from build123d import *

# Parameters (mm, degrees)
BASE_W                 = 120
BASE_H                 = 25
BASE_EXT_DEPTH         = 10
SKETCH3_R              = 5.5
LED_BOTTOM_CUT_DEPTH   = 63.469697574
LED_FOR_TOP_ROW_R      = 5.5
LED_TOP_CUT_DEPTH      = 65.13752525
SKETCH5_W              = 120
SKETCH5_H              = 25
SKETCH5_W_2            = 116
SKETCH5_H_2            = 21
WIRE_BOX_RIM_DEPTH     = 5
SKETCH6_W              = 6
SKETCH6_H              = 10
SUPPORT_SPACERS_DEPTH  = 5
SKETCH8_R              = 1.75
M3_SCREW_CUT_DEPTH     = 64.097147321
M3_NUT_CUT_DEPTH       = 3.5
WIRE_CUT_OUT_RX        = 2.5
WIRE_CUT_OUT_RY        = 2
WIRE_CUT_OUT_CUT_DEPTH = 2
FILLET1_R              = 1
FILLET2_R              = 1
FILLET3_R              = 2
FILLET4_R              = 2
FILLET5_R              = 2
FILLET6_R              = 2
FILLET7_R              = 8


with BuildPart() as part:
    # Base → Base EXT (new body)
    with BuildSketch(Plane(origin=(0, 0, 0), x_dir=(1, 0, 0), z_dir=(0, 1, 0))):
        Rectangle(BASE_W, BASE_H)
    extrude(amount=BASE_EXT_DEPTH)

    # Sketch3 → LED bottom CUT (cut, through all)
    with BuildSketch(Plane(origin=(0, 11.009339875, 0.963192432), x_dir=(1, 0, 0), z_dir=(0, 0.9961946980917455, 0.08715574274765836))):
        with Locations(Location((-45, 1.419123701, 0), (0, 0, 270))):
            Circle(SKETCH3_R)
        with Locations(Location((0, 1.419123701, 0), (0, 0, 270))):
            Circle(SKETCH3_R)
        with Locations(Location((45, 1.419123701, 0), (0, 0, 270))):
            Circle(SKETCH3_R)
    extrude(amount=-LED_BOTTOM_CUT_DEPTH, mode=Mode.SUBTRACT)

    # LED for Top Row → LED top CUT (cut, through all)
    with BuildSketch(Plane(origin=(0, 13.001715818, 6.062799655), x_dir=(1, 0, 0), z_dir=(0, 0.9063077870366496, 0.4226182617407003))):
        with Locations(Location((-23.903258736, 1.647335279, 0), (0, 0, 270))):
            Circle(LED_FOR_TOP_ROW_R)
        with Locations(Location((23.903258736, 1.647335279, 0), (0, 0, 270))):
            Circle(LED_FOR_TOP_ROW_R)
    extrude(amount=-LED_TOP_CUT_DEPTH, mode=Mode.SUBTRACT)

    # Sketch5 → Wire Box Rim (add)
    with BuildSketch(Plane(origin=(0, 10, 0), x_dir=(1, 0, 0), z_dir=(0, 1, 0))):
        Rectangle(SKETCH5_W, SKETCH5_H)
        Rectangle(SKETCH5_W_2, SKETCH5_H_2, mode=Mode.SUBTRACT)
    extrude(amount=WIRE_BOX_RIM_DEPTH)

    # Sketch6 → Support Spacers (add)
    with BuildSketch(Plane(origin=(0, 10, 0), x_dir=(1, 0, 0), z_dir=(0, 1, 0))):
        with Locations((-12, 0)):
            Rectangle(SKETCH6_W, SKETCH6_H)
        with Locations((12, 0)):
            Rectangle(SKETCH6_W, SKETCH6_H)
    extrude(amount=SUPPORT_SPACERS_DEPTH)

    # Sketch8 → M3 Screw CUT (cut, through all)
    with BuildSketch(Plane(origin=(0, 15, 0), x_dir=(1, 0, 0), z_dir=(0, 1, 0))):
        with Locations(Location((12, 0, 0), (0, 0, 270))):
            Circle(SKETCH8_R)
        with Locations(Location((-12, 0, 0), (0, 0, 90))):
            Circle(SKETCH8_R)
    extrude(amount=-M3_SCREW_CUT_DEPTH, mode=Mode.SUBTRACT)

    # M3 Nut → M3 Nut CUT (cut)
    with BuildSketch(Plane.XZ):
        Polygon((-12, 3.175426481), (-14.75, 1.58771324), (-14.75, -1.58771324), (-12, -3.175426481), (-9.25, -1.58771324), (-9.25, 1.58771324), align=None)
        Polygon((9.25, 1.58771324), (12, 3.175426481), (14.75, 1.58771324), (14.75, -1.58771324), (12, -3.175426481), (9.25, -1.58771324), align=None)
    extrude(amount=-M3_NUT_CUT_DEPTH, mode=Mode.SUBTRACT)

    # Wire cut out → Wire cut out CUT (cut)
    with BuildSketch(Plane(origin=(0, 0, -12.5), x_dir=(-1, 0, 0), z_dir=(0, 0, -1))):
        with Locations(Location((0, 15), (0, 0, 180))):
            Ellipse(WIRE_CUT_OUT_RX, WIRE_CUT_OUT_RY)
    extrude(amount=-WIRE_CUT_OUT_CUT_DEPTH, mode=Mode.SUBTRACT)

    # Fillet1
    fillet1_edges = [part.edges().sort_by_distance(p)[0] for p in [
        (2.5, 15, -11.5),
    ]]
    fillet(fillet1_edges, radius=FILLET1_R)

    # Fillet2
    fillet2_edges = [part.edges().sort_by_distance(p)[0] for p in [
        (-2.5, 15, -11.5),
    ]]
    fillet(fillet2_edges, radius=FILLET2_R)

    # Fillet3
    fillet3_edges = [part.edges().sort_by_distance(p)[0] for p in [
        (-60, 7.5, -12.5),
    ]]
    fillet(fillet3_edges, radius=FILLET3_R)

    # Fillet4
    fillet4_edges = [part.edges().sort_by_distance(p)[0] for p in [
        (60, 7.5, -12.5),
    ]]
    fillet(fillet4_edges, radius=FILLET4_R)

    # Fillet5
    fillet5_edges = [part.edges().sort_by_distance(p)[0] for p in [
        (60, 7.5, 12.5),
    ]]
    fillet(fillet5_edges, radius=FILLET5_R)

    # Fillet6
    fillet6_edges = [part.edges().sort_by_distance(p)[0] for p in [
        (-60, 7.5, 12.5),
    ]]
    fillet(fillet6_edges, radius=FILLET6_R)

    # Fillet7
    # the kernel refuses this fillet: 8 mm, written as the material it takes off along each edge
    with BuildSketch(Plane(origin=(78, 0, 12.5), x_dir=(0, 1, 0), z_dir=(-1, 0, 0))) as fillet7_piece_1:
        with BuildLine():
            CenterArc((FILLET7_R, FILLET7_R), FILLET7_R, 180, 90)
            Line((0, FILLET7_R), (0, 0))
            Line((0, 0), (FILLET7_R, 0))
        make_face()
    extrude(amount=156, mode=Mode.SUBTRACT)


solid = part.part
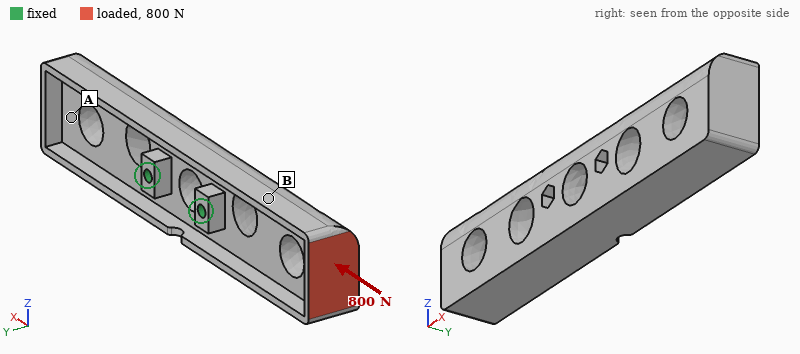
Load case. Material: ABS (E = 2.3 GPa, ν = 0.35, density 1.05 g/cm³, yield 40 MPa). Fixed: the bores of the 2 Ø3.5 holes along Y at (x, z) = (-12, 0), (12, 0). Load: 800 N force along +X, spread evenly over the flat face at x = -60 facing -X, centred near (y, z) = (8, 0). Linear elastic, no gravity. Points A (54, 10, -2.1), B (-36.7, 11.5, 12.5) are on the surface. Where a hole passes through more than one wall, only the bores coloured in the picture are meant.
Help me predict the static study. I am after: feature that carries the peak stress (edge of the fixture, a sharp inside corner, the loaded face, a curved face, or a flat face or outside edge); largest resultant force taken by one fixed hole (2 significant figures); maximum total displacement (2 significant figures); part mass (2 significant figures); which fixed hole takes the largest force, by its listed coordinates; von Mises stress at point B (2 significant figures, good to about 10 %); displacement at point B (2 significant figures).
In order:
the loaded face
560 N
0.65 mm
28 g
(-12, 0)
8.7 MPa
0.16 mm
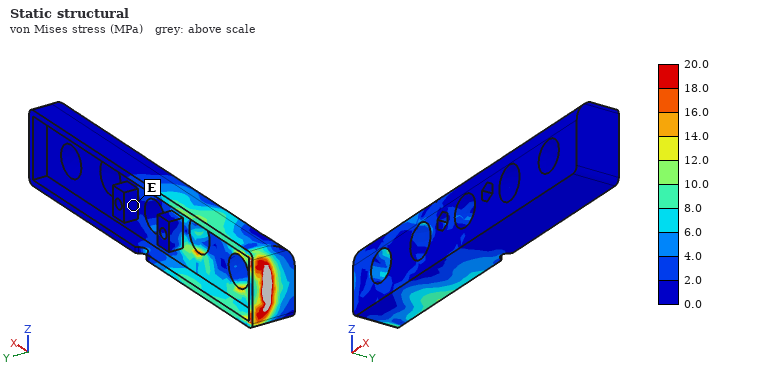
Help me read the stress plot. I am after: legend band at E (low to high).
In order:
0.0 to 2.0 MPa
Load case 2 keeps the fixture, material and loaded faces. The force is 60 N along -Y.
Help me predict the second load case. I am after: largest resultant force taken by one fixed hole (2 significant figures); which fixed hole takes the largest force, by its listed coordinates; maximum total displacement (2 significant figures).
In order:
130 N
(-12, 0)
0.66 mm
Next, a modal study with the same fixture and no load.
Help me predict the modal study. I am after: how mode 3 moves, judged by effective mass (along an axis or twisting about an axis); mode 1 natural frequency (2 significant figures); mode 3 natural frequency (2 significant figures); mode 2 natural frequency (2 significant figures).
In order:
twisting about Y
840 Hz
1200 Hz
860 Hz
